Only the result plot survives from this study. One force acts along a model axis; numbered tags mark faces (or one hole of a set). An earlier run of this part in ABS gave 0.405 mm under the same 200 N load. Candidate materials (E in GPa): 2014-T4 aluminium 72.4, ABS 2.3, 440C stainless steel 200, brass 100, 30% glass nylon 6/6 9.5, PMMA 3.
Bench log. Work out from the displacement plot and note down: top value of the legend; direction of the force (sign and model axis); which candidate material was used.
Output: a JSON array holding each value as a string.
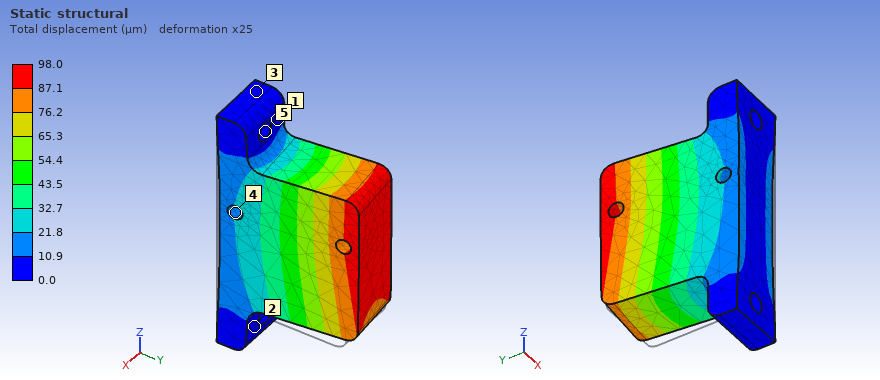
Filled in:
["98.0 µm", "-X", "30% glass nylon 6/6"]
